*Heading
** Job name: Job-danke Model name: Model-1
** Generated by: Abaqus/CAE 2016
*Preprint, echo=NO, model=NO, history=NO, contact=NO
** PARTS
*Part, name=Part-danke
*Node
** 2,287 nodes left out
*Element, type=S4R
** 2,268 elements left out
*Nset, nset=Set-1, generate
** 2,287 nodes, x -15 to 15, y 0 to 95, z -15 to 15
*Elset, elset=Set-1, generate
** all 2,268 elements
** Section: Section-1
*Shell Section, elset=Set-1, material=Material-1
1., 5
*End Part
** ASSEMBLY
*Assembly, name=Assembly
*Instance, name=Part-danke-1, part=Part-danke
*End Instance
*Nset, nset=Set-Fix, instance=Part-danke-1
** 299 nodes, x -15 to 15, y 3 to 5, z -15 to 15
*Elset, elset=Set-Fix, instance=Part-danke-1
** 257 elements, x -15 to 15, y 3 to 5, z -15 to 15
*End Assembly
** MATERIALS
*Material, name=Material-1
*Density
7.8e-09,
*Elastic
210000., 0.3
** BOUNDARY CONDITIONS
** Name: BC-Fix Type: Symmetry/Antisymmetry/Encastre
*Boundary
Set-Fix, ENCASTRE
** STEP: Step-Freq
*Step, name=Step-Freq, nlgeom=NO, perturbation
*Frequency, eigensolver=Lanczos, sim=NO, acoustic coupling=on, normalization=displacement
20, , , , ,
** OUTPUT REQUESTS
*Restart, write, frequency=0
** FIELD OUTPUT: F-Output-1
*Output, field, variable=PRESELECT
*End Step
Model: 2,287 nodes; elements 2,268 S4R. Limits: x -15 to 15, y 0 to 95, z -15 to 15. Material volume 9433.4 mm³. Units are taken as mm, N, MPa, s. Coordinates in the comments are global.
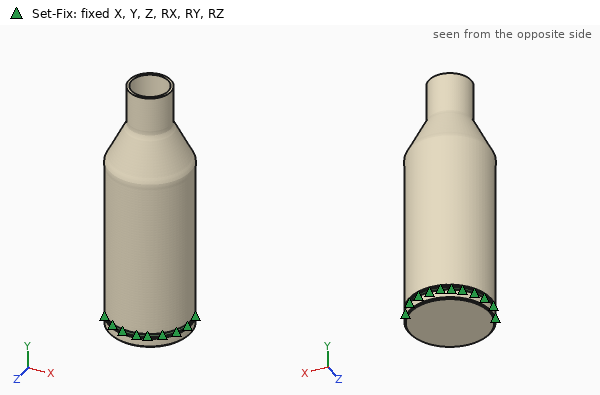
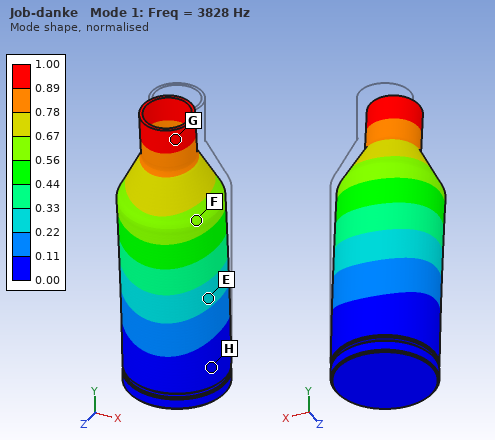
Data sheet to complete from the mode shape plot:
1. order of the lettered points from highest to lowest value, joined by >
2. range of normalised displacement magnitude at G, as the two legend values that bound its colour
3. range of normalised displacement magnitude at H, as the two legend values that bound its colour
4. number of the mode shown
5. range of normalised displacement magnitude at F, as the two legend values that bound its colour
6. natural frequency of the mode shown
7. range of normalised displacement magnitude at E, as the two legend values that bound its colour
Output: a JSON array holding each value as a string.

["G > F > E > H", "0.89 to 1.00", "0.00 to 0.11", "1", "0.56 to 0.67", "3828 Hz", "0.22 to 0.33"]
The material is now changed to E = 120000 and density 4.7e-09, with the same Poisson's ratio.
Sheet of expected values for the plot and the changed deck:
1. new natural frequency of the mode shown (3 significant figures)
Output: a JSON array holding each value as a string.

["3730 Hz"]
